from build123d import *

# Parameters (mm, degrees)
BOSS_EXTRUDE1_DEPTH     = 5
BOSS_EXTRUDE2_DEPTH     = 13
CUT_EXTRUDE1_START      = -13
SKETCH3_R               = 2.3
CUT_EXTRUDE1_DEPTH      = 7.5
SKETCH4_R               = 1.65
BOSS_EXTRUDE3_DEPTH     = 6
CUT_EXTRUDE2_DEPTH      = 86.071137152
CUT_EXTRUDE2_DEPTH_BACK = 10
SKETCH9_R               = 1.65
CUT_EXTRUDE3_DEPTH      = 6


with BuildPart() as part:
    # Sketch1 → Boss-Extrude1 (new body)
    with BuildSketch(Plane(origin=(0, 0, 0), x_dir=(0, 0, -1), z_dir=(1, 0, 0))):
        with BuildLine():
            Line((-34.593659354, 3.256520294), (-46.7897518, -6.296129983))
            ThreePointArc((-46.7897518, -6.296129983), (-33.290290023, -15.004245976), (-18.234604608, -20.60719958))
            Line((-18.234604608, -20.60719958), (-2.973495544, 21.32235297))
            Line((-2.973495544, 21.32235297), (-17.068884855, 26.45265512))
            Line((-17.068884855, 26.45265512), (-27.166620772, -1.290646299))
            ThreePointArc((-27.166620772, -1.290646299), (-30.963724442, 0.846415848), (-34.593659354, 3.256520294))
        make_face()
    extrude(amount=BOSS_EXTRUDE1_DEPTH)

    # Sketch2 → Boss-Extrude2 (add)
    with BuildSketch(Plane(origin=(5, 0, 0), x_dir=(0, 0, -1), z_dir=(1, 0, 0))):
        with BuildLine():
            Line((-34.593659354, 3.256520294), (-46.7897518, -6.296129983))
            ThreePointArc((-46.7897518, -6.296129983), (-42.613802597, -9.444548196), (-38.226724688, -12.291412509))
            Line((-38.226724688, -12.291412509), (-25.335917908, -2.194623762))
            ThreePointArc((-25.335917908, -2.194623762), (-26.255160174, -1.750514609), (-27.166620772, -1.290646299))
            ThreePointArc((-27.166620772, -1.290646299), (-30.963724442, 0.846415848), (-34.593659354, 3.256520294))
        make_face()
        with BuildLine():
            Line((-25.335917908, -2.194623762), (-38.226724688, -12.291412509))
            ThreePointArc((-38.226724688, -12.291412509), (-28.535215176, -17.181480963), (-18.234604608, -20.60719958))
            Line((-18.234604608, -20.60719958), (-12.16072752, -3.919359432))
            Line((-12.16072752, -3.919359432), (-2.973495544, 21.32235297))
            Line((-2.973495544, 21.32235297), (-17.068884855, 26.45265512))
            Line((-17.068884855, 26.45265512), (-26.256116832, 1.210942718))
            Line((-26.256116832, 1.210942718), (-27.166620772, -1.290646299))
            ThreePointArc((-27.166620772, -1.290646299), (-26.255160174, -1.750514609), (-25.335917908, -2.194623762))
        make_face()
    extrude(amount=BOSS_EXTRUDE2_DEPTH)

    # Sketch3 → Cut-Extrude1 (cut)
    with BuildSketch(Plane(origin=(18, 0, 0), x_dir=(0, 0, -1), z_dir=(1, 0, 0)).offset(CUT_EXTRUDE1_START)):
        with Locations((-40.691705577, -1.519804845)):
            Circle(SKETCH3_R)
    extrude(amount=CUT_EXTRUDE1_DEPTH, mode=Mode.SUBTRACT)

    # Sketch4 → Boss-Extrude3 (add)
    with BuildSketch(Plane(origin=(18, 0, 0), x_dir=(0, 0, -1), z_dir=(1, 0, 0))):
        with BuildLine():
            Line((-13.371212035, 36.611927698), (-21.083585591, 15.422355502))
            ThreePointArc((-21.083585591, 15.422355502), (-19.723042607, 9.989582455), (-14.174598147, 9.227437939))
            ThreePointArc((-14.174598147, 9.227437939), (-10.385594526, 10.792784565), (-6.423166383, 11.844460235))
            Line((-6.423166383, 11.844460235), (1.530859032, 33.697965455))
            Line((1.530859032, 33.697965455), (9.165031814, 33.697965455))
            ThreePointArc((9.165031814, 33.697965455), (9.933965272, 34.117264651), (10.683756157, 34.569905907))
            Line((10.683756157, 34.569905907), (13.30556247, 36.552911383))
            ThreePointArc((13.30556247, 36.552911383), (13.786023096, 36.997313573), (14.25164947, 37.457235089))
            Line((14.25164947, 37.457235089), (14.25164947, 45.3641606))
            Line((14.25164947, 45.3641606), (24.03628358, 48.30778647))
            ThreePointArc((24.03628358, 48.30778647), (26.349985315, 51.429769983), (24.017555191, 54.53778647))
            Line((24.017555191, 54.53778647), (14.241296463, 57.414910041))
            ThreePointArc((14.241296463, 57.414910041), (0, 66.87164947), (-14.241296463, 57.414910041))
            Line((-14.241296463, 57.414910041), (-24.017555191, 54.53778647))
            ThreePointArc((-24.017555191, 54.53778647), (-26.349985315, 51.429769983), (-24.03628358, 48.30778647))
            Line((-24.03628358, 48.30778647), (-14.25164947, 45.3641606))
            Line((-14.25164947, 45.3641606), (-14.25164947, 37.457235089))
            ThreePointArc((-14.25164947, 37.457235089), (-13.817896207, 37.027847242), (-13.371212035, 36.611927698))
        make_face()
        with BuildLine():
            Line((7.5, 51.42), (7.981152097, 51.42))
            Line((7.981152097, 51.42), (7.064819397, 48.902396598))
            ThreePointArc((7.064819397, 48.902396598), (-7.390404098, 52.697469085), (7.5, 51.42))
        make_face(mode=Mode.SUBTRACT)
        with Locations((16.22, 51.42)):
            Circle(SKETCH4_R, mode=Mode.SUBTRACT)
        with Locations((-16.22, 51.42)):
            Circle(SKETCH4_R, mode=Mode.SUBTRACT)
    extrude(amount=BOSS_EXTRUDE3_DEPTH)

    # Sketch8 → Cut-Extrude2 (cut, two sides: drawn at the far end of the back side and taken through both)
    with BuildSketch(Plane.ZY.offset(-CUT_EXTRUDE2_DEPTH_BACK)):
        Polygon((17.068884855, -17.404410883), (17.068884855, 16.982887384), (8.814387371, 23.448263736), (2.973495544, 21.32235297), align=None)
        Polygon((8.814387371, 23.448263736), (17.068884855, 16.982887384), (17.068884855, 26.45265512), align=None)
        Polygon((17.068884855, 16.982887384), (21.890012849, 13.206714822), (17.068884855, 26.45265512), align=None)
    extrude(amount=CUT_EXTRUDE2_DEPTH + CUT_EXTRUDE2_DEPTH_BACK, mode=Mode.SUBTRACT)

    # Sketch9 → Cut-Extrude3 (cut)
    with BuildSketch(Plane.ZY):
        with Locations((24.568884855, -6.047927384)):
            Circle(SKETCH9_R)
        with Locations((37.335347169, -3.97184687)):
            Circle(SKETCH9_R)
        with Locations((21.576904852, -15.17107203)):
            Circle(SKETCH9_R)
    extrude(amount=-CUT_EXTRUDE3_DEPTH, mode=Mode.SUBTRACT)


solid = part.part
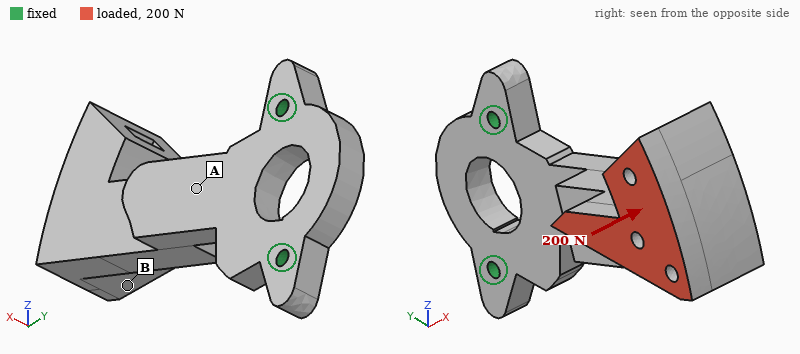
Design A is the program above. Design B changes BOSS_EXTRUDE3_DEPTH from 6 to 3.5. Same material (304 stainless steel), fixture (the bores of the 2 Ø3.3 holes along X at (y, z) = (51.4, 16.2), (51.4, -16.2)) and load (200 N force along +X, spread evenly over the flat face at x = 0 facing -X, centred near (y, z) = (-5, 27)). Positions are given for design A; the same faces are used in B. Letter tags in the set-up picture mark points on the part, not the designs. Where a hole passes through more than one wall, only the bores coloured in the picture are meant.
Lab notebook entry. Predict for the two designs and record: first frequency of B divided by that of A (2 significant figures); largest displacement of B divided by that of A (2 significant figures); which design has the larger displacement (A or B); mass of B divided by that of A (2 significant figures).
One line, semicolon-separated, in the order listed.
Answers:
0.48; 4.5; B; 0.84
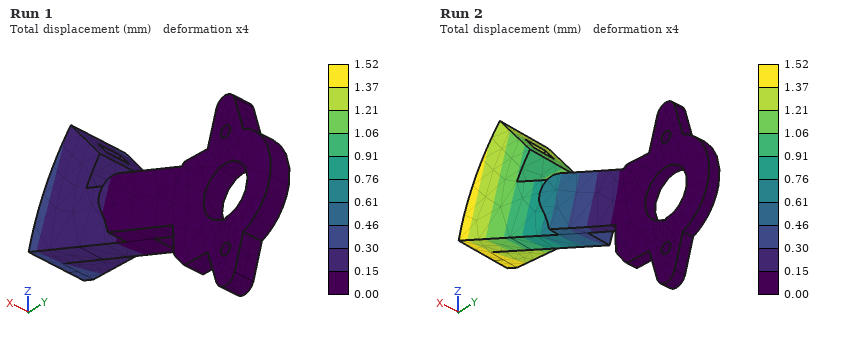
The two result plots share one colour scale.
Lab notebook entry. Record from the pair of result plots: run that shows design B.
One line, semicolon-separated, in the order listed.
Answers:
Run 2
